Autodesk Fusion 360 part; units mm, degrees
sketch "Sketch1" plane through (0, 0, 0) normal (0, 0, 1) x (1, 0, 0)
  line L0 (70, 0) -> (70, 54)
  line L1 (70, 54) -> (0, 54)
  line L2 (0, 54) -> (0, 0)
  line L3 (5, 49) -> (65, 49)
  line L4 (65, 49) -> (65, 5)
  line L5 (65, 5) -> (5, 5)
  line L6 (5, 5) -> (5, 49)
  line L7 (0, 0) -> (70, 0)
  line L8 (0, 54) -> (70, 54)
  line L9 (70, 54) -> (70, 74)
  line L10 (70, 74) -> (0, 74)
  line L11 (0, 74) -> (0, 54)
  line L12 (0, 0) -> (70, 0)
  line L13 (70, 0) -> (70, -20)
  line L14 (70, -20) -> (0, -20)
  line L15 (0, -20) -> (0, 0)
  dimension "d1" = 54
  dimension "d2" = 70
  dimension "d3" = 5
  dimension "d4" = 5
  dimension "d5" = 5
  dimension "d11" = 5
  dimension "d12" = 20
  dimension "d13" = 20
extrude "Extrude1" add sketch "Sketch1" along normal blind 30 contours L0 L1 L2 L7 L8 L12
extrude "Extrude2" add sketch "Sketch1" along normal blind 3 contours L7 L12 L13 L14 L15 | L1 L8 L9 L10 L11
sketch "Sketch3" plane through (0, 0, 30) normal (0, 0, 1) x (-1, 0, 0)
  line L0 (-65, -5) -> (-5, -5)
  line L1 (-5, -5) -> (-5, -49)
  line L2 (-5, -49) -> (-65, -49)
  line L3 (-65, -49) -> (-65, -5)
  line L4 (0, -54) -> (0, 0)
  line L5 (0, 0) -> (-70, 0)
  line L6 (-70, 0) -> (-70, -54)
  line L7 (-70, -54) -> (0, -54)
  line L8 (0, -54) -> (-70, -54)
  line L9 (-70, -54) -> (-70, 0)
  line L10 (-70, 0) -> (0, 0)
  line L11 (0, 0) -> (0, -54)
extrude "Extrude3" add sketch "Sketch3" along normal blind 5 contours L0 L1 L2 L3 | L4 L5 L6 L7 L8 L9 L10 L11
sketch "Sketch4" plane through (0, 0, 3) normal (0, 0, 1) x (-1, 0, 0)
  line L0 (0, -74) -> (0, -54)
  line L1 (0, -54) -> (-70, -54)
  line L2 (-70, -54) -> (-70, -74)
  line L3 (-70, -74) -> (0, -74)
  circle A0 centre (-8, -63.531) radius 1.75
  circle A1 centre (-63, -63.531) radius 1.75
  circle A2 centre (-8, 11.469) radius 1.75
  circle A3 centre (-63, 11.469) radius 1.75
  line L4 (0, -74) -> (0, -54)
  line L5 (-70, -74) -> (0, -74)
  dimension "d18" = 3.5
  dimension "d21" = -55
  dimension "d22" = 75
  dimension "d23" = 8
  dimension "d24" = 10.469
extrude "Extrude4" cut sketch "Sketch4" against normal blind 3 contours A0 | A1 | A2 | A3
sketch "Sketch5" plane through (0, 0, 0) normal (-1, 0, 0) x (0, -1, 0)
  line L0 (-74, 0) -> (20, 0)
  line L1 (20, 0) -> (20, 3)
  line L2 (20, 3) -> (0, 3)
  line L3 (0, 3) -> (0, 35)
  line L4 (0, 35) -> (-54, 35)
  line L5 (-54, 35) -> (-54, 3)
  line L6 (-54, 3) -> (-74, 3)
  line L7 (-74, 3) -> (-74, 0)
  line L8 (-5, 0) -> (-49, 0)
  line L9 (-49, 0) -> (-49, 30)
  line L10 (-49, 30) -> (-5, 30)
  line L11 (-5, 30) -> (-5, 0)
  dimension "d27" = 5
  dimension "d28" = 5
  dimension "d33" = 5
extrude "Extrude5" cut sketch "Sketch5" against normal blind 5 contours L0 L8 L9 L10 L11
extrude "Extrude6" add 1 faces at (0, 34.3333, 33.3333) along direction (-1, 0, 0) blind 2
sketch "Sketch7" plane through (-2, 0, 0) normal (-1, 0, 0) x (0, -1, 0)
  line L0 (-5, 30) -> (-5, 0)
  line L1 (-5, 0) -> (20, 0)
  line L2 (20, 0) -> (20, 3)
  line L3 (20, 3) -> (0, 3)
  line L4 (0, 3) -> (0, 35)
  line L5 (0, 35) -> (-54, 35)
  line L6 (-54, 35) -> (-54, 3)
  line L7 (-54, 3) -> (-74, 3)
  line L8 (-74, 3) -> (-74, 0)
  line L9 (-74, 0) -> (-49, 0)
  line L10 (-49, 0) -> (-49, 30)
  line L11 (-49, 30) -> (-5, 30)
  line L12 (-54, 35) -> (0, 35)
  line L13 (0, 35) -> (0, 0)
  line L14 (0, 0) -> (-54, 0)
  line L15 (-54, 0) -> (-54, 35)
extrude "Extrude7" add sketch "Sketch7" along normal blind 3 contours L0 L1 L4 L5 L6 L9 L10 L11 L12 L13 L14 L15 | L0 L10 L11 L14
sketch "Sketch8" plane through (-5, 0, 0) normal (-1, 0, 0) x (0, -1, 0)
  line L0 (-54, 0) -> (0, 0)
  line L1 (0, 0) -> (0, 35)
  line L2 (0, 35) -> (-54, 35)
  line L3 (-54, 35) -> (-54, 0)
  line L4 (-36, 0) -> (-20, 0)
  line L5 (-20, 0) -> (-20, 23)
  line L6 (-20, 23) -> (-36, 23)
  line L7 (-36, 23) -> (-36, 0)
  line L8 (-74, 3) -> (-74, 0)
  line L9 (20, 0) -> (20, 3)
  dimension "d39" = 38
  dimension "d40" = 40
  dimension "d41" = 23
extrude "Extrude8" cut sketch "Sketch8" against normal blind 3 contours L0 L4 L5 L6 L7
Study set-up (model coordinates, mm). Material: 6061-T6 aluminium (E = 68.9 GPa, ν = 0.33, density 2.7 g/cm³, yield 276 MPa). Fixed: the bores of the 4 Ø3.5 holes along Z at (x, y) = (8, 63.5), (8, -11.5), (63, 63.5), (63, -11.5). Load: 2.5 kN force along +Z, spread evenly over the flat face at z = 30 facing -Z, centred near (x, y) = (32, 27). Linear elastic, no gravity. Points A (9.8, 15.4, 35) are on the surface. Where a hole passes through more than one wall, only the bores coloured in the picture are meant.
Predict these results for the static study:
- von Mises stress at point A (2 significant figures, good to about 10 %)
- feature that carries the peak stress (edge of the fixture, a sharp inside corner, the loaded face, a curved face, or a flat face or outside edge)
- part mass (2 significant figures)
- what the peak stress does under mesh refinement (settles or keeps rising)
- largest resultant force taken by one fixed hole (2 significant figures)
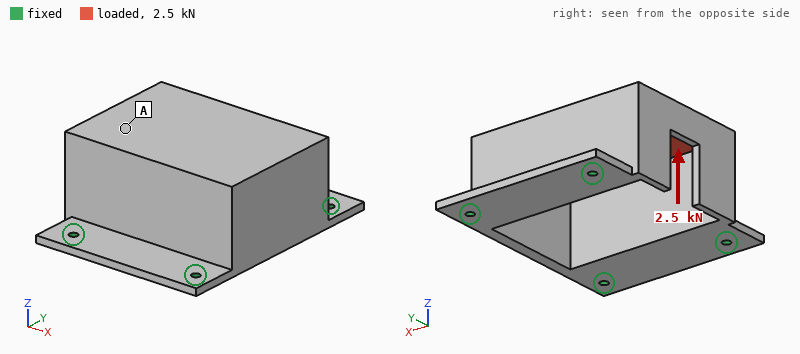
12 MPa
edge of the fixture
160 g
keeps rising
830 N
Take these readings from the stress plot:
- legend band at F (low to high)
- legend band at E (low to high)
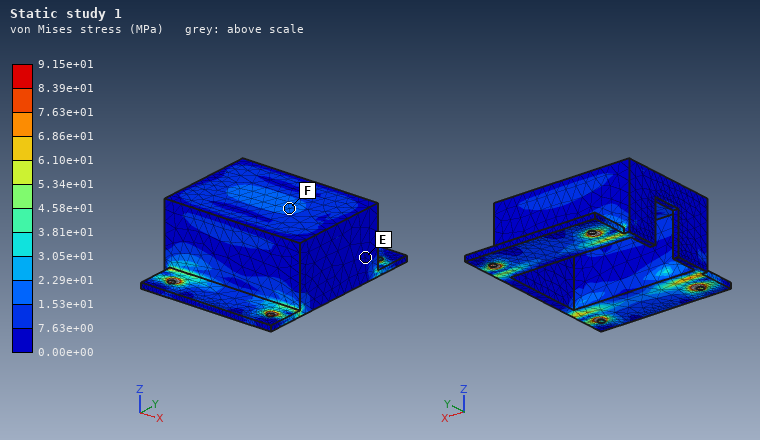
1.53e+01 to 2.29e+01 MPa
0.00e+00 to 7.63e+00 MPa
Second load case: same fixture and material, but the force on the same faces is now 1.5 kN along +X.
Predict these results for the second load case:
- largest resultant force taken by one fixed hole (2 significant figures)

670 N
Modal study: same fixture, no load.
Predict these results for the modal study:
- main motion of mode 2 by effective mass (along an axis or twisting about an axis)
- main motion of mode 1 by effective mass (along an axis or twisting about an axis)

along Z
along X
